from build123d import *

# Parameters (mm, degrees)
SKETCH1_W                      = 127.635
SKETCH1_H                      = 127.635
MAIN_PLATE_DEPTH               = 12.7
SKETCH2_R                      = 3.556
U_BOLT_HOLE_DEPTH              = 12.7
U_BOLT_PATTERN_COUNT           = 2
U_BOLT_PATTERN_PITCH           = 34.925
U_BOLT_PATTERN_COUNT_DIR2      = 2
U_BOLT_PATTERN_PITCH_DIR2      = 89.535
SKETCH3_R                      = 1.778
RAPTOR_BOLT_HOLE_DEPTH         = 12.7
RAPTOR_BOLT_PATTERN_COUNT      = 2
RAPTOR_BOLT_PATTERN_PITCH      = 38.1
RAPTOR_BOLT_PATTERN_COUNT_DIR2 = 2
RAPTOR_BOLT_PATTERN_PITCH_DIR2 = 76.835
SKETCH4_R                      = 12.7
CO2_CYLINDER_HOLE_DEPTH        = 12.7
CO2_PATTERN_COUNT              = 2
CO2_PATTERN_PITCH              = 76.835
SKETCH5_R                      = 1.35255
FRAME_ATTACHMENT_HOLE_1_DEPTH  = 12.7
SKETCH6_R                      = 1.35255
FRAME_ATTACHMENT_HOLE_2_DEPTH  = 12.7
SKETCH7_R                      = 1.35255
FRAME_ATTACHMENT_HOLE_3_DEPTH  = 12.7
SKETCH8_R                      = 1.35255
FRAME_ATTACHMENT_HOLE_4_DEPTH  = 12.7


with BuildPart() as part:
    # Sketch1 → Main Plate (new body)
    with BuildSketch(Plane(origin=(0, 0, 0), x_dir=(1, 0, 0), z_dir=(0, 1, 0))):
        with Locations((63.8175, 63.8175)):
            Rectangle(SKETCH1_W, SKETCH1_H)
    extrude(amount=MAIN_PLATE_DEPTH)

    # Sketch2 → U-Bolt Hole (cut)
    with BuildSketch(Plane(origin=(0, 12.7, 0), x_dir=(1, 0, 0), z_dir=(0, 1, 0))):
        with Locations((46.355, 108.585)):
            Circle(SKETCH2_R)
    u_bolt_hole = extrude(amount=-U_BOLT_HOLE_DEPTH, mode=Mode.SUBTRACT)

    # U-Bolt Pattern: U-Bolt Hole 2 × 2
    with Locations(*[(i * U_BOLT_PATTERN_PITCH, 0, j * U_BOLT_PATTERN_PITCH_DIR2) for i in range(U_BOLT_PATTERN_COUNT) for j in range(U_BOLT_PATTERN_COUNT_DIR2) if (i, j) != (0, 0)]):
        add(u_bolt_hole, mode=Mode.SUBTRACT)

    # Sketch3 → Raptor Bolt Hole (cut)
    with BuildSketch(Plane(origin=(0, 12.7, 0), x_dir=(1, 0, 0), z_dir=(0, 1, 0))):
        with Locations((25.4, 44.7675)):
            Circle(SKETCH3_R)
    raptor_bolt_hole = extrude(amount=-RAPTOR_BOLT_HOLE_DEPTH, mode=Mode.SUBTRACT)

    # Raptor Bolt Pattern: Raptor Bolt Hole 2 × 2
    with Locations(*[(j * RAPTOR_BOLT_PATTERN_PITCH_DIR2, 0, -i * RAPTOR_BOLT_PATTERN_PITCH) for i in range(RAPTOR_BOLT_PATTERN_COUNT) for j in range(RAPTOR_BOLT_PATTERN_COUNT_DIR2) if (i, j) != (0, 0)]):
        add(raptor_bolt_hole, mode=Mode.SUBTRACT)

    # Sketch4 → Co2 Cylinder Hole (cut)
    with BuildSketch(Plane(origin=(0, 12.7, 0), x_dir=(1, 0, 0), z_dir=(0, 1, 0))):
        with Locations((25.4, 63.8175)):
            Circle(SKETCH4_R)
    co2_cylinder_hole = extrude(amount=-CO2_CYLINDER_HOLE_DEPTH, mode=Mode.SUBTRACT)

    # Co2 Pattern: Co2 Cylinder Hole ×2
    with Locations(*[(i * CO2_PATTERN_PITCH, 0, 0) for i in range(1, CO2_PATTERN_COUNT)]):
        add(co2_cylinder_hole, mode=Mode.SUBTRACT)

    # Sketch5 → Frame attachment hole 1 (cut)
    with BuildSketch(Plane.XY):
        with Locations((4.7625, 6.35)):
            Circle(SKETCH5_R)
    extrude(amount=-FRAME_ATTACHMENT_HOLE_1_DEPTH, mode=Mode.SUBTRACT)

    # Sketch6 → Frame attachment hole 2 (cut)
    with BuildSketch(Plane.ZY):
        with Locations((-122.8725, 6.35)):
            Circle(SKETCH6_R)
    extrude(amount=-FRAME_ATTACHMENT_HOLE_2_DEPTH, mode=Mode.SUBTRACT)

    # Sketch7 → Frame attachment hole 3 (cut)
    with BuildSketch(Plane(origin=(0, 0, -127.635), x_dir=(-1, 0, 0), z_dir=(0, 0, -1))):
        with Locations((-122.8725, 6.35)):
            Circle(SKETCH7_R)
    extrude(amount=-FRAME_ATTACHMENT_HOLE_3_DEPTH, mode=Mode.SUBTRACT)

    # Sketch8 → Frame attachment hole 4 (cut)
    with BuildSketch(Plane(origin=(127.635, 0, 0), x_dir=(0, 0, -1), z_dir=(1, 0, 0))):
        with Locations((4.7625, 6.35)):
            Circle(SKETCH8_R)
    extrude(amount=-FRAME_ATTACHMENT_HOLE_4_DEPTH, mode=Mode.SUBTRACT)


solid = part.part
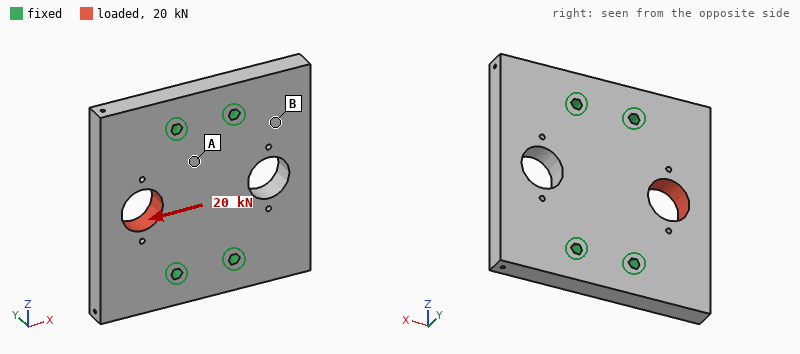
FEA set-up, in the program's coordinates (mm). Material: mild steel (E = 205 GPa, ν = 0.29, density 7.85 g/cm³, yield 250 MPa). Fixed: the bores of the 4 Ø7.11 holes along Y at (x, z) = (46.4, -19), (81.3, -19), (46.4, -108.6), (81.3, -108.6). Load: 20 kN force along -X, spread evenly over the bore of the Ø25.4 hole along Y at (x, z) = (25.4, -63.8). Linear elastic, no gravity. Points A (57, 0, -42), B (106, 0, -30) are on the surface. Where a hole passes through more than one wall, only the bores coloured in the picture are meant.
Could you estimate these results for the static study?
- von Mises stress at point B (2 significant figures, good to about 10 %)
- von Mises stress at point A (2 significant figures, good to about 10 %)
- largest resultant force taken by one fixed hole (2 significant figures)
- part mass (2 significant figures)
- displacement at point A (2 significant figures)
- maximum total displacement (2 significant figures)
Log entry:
5.6 MPa
17 MPa
6.2 kN
1.5 kg
2.9 µm
10 µm
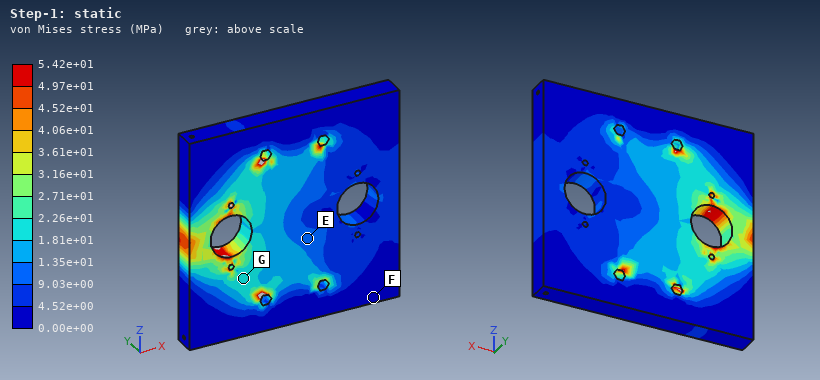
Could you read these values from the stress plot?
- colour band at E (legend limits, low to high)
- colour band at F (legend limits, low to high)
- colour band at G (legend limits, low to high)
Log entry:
9.03e+00 to 1.35e+01 MPa
0.00e+00 to 4.52e+00 MPa
1.81e+01 to 2.26e+01 MPa
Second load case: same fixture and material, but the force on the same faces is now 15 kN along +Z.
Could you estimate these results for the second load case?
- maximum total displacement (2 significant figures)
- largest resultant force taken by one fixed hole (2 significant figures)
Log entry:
7.8 µm
7.2 kN
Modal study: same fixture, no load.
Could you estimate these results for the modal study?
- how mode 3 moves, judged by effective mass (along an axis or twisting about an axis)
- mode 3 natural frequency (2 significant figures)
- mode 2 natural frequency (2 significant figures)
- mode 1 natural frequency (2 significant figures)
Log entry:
twisting about X
5400 Hz
3800 Hz
3600 Hz
